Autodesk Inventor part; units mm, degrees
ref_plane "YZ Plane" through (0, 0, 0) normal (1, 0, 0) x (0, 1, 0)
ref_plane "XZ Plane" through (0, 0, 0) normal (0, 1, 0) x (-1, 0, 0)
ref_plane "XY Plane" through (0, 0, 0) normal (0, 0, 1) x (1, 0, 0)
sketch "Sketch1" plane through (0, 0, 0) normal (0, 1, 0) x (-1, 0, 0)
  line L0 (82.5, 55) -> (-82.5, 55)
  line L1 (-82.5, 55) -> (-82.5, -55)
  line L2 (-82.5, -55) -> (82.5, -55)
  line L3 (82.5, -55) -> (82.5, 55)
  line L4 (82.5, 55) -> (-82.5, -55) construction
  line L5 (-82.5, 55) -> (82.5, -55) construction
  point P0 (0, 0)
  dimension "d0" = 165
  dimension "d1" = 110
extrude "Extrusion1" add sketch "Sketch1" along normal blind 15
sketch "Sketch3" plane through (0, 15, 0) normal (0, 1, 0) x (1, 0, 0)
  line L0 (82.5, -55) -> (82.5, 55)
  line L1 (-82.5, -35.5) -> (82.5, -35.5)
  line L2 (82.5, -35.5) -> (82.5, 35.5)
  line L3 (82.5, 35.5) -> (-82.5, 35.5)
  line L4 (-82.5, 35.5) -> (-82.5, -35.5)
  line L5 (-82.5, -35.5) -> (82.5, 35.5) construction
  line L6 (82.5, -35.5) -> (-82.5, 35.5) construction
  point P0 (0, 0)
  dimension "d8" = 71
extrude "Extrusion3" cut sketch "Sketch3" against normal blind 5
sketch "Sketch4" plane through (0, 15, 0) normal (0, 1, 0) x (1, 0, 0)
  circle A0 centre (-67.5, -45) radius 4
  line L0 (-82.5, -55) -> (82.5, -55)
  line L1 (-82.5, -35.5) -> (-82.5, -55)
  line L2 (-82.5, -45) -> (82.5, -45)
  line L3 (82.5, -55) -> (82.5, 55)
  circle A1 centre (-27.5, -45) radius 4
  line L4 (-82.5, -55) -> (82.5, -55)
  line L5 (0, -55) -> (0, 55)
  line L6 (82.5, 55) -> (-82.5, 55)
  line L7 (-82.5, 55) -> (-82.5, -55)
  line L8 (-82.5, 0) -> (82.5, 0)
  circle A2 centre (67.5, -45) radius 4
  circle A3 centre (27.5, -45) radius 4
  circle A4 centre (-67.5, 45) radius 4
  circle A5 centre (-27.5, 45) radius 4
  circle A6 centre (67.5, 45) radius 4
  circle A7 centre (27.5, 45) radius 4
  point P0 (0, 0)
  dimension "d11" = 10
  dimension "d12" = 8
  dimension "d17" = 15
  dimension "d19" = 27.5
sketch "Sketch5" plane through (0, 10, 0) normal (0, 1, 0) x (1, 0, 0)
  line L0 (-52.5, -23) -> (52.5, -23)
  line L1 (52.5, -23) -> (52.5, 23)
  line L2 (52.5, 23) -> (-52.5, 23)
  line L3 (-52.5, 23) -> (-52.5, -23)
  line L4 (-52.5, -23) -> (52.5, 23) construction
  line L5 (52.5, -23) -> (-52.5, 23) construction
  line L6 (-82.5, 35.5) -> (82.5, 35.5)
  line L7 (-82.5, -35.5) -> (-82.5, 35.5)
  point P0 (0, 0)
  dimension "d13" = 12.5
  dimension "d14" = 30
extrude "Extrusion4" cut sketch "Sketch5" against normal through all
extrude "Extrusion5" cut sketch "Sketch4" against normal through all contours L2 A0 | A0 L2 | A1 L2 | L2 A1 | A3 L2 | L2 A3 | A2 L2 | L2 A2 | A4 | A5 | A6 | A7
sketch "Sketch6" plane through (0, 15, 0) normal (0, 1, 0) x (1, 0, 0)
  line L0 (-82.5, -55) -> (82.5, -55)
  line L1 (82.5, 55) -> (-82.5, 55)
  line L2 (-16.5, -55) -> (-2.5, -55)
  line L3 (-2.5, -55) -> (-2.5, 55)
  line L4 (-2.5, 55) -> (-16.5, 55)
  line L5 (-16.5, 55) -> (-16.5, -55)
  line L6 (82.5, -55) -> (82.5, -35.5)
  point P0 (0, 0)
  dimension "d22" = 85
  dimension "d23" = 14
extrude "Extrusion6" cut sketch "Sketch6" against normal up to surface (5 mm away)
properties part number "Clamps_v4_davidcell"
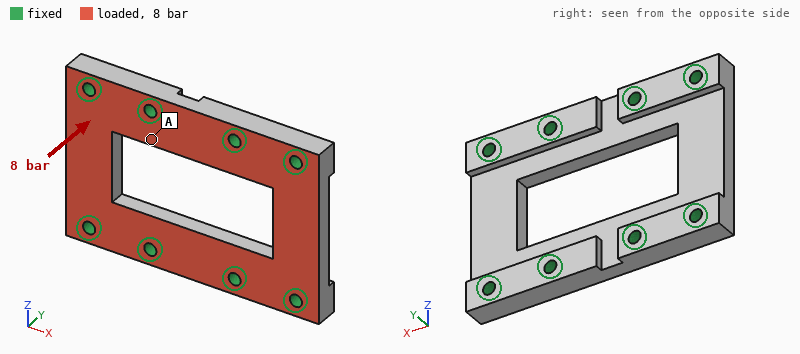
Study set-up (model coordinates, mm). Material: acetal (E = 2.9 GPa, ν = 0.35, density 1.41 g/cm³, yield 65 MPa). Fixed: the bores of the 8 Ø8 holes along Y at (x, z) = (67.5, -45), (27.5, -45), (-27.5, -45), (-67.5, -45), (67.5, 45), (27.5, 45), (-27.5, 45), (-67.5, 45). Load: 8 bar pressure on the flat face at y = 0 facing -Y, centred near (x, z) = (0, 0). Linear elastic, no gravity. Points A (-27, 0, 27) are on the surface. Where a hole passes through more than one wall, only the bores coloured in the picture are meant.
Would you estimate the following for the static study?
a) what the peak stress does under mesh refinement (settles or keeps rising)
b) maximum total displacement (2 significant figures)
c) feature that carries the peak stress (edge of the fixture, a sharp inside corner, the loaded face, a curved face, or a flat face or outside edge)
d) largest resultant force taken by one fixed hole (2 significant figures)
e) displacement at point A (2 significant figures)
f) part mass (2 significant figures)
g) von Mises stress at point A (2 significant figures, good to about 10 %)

keeps rising
0.45 mm
edge of the fixture
1.4 kN
0.084 mm
220 g
3.7 MPa
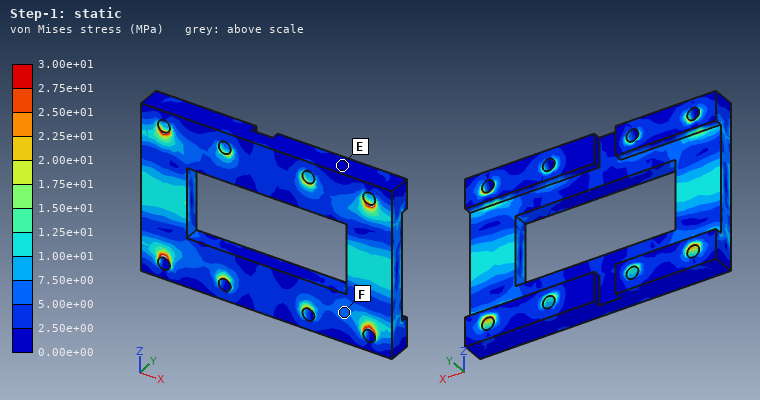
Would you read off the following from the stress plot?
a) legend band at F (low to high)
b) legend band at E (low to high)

5.00e+00 to 7.50e+00 MPa
0.00e+00 to 2.50e+00 MPa
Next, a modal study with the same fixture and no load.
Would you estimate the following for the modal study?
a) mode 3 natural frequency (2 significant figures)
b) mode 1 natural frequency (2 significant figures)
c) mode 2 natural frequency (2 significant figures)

3800 Hz
2200 Hz
2200 Hz
